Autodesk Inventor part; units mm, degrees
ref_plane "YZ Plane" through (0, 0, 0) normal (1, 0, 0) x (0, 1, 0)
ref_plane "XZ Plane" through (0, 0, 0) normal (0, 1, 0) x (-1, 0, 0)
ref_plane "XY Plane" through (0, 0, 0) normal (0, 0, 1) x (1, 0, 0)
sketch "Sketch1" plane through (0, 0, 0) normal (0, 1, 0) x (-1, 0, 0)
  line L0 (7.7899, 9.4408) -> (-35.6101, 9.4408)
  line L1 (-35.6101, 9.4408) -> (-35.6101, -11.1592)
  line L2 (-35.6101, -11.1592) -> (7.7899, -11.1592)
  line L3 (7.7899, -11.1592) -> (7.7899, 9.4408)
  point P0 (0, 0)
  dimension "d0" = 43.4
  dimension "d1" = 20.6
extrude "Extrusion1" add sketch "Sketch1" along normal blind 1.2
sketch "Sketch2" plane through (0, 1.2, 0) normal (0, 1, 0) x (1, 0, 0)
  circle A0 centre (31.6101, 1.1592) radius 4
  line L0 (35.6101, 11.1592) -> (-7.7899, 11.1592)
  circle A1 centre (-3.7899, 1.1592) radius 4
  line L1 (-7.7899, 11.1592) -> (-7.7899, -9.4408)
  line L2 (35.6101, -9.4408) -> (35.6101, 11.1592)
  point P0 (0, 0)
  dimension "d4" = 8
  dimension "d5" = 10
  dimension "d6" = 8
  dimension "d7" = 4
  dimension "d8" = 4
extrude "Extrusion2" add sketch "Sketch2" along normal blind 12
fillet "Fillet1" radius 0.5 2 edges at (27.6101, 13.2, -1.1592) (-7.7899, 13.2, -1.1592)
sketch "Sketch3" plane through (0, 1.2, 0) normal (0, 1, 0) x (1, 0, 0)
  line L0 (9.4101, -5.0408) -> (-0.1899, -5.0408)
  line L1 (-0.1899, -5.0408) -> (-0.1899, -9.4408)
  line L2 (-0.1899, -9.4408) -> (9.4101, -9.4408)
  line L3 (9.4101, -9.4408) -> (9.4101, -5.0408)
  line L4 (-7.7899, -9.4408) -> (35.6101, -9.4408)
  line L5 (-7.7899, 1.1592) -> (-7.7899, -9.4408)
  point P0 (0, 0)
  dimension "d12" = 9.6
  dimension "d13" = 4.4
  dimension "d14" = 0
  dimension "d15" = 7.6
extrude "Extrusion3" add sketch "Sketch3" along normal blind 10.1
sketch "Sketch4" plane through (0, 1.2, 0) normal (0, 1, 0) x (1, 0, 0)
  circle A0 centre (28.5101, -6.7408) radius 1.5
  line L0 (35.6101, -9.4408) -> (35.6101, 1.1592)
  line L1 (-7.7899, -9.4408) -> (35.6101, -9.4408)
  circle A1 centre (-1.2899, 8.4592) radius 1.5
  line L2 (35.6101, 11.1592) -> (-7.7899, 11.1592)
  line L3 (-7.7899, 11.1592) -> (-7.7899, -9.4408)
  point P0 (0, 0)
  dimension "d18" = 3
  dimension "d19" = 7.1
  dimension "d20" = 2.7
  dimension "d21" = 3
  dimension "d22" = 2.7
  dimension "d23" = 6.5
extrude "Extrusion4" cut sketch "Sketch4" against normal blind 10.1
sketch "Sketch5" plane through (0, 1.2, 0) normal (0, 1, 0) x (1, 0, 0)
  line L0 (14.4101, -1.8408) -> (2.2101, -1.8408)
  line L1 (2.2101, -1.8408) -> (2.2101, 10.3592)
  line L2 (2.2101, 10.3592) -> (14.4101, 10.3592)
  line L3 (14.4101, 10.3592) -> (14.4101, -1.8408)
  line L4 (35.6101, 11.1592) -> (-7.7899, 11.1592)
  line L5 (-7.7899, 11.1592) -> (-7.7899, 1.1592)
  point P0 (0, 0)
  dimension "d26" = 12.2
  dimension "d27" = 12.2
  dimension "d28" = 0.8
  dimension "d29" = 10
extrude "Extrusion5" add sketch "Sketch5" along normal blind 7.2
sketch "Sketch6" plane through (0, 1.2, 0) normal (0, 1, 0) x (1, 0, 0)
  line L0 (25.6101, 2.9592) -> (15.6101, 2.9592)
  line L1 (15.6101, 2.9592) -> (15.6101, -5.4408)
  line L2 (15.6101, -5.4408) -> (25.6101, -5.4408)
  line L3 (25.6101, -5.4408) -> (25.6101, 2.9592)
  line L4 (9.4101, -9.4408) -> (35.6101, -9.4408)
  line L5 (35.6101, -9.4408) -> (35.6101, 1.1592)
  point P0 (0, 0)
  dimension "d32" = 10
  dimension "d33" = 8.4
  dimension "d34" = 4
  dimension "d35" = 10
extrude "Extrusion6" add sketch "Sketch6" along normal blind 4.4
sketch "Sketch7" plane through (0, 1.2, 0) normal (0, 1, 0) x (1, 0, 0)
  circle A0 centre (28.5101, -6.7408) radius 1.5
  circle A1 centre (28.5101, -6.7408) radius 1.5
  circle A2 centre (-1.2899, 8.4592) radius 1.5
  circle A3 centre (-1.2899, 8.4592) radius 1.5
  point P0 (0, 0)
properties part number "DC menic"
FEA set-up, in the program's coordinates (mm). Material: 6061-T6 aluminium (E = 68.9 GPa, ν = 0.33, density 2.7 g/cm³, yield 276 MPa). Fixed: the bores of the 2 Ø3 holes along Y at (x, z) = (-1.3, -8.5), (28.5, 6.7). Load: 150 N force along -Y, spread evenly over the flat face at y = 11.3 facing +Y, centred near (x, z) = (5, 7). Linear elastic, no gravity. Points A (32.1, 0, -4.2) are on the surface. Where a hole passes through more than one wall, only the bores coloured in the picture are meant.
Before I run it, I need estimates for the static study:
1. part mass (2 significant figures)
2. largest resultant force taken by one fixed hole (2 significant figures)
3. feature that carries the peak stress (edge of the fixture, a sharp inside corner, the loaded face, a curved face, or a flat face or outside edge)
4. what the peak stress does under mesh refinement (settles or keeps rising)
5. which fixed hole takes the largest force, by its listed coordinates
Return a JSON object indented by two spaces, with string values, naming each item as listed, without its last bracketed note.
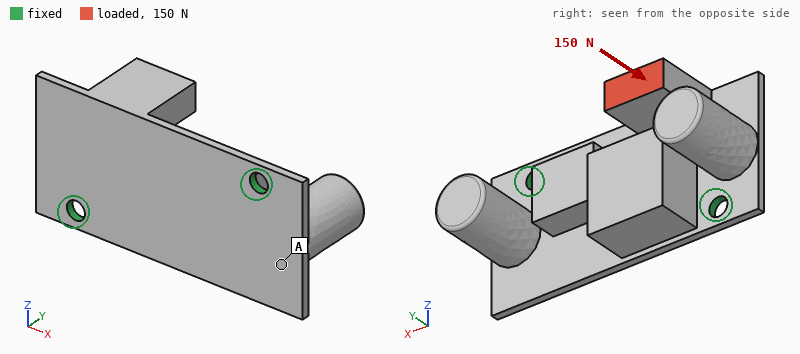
{
  "part mass": "11 g",
  "largest resultant force taken by one fixed hole": "120 N",
  "feature that carries the peak stress": "edge of the fixture",
  "what the peak stress does under mesh refinement": "keeps rising",
  "which fixed hole takes the largest force, by its listed coordinates": "(-1.3, -8.5)"
}
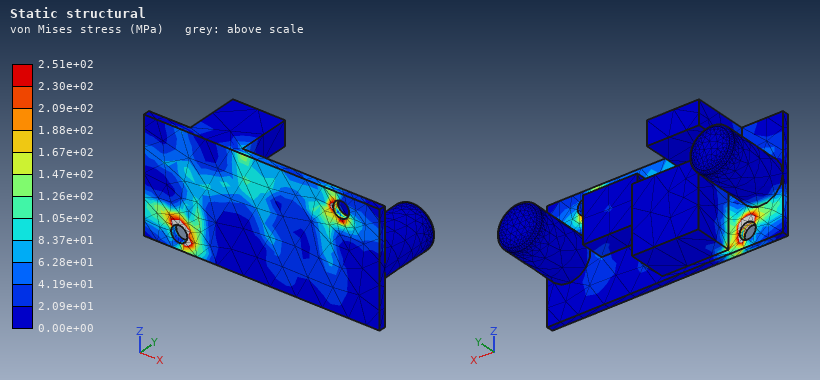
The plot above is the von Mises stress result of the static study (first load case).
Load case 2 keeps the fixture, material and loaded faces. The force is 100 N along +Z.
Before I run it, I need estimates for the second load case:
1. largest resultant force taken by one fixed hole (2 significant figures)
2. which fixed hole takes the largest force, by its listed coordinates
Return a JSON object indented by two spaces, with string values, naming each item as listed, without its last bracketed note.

{
  "largest resultant force taken by one fixed hole": "77 N",
  "which fixed hole takes the largest force, by its listed coordinates": "(-1.3, -8.5)"
}
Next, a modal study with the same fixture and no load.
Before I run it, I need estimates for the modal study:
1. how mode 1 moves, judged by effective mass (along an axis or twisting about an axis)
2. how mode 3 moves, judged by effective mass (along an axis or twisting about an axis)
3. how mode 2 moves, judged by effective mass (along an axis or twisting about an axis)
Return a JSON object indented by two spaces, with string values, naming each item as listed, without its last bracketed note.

{
  "how mode 1 moves, judged by effective mass": "along Z",
  "how mode 3 moves, judged by effective mass": "along Y",
  "how mode 2 moves, judged by effective mass": "along Y"
}
